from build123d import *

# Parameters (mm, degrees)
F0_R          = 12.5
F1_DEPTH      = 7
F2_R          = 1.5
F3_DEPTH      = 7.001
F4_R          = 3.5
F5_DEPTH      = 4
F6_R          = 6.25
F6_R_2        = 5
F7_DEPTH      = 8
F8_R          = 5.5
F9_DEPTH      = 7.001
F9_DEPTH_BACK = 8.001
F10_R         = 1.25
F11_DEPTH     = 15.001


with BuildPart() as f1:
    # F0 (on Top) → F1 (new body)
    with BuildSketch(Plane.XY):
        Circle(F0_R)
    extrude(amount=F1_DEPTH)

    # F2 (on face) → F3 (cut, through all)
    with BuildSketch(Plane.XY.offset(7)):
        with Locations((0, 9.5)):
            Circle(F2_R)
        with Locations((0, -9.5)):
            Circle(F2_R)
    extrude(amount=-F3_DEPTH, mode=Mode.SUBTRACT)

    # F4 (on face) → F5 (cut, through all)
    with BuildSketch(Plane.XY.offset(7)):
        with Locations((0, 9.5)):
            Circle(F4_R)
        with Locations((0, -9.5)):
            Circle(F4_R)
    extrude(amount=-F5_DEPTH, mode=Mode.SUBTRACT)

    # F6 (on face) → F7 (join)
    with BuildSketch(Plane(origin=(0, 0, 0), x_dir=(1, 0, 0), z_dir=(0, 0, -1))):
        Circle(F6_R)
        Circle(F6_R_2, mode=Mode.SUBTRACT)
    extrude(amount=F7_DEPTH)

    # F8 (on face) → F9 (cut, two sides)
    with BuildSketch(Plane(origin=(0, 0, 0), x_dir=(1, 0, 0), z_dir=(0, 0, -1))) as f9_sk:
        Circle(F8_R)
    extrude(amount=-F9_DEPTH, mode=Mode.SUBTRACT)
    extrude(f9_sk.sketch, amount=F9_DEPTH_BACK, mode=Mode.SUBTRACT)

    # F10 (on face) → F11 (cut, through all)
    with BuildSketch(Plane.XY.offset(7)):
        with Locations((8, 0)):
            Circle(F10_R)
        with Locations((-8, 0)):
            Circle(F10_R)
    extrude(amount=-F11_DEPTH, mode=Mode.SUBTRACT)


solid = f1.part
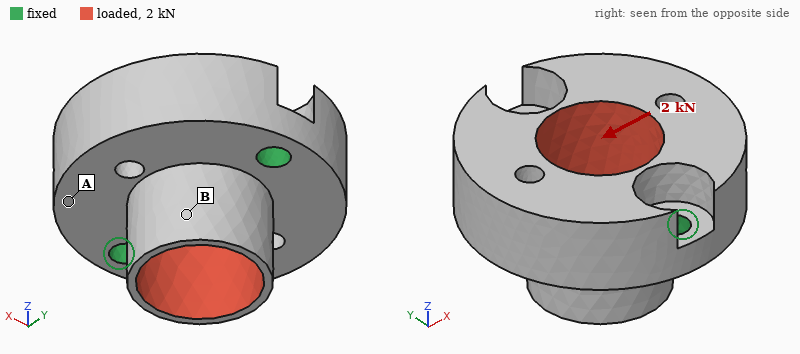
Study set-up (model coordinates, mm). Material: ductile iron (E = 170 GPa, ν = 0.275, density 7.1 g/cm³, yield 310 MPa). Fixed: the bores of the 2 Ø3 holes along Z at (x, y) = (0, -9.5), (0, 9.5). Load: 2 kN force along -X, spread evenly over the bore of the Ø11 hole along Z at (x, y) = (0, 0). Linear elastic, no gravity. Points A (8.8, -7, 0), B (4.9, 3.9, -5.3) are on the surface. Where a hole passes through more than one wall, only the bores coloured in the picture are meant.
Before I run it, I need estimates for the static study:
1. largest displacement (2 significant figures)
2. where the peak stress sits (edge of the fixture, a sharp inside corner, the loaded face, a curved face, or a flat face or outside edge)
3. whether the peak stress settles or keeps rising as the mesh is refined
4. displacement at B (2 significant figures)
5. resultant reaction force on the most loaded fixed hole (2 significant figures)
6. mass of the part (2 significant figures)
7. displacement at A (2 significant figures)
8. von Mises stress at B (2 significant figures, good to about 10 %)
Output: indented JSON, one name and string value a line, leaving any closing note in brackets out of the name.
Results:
{
  "largest displacement": "16 µm",
  "where the peak stress sits": "edge of the fixture",
  "whether the peak stress settles or keeps rising as the mesh is refined": "keeps rising",
  "displacement at B": "12 µm",
  "resultant reaction force on the most loaded fixed hole": "1.0 kN",
  "mass of the part": "18 g",
  "displacement at A": "5.5 µm",
  "von Mises stress at B": "35 MPa"
}
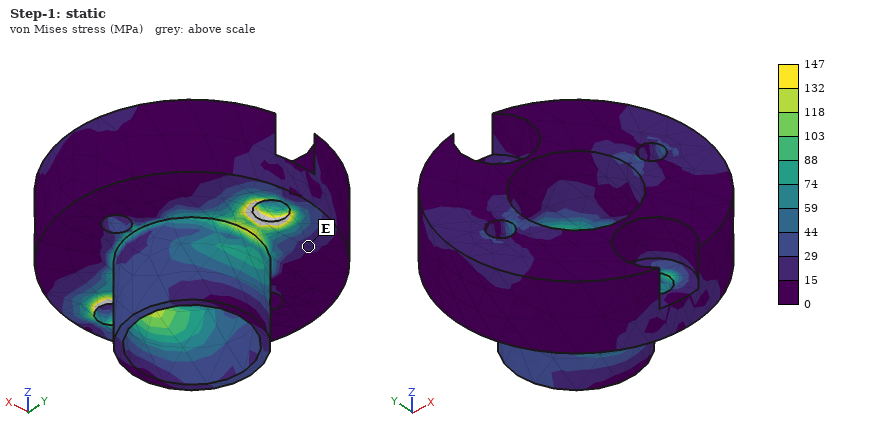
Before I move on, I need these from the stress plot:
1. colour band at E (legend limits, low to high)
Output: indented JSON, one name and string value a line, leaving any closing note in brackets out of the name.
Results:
{
  "colour band at E": "15 to 29 MPa"
}
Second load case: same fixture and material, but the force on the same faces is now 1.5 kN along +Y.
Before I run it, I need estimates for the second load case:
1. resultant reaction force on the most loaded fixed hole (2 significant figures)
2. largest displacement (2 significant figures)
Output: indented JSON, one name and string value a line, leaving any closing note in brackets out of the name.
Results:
{
  "resultant reaction force on the most loaded fixed hole": "780 N",
  "largest displacement": "7.4 µm"
}
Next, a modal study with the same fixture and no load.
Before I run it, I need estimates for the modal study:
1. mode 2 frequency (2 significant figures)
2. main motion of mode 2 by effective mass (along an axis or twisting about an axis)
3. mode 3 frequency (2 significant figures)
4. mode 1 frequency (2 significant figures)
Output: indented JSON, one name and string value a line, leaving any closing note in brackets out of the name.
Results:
{
  "mode 2 frequency": "19 kHz",
  "main motion of mode 2 by effective mass": "along Z",
  "mode 3 frequency": "31 kHz",
  "mode 1 frequency": "11 kHz"
}
